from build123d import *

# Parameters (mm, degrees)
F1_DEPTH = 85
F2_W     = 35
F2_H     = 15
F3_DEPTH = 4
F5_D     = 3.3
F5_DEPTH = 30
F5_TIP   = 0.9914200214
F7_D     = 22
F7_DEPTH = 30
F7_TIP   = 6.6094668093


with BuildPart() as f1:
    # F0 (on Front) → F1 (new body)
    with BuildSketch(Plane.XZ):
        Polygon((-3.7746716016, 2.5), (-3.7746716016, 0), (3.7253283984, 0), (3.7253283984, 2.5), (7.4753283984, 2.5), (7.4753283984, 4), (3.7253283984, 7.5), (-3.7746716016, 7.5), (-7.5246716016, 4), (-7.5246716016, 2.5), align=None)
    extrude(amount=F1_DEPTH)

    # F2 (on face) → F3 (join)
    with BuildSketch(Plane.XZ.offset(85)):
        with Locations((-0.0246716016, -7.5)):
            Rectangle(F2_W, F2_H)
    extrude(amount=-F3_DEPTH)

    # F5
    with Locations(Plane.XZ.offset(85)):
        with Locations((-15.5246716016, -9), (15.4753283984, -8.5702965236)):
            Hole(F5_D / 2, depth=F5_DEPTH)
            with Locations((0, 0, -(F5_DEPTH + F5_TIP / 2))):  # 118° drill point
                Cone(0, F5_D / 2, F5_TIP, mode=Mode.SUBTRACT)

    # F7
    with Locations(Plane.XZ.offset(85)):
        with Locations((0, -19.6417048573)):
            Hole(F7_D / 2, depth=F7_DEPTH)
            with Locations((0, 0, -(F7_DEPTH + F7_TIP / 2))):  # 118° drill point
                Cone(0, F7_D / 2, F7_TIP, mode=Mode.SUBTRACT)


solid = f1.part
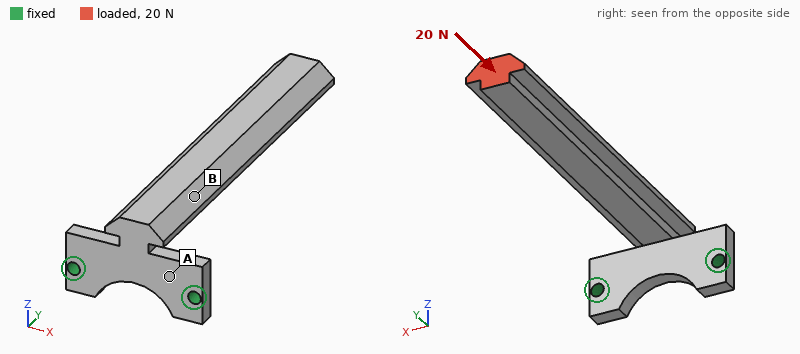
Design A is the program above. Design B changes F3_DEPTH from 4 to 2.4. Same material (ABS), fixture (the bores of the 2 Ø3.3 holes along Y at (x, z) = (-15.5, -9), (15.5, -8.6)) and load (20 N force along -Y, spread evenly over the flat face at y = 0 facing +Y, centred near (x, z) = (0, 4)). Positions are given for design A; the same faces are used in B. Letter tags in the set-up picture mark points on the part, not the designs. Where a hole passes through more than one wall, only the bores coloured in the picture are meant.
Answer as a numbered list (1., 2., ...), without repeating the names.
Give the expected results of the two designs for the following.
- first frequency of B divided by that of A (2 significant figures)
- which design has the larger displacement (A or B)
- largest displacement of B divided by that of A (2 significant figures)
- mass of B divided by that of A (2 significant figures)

1. 0.55
2. B
3. 3.9
4. 0.92
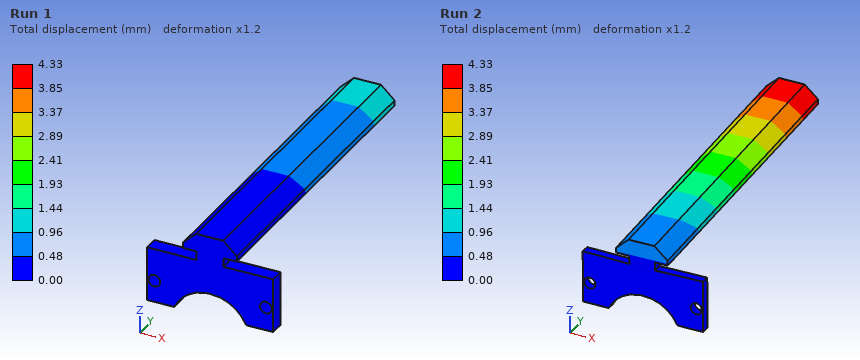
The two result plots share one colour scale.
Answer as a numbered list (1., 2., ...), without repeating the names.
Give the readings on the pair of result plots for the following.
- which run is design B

1. Run 2
